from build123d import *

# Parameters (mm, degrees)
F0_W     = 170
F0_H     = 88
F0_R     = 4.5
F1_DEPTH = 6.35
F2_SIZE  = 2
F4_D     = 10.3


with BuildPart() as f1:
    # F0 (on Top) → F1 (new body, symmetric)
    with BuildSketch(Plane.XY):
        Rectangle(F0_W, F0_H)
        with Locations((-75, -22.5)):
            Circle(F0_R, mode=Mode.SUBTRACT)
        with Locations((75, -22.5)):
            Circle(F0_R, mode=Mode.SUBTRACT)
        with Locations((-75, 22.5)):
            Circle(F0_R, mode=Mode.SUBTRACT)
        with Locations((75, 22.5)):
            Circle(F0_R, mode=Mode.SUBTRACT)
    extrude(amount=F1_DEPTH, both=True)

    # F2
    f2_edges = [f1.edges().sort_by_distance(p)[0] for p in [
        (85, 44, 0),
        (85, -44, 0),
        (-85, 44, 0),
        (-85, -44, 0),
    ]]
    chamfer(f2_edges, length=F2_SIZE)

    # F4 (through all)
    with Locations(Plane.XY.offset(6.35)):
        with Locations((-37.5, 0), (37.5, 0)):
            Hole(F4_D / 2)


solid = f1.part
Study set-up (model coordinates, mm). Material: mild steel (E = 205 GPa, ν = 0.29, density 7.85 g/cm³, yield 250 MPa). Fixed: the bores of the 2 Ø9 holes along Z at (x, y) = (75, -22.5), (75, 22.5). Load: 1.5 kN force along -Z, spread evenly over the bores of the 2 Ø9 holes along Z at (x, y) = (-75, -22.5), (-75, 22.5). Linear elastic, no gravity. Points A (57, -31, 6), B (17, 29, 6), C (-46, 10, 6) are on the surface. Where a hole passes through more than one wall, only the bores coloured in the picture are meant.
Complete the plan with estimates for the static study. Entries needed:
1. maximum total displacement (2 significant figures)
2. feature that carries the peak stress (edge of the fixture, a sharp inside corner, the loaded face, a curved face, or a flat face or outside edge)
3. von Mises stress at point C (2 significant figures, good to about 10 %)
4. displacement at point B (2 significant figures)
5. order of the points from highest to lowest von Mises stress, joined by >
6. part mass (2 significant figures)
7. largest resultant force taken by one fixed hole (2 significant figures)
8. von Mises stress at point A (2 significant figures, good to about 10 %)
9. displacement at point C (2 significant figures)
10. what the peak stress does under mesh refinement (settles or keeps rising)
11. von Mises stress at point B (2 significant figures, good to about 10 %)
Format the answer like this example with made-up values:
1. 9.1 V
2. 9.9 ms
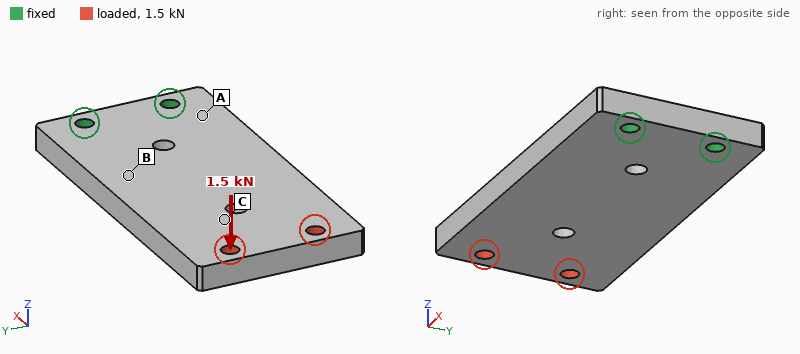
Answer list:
1. 0.63 mm
2. edge of the fixture
3. 21 MPa
4. 0.12 mm
5. A > B > C
6. 1.4 kg
7. 750 N
8. 82 MPa
9. 0.41 mm
10. keeps rising
11. 59 MPa
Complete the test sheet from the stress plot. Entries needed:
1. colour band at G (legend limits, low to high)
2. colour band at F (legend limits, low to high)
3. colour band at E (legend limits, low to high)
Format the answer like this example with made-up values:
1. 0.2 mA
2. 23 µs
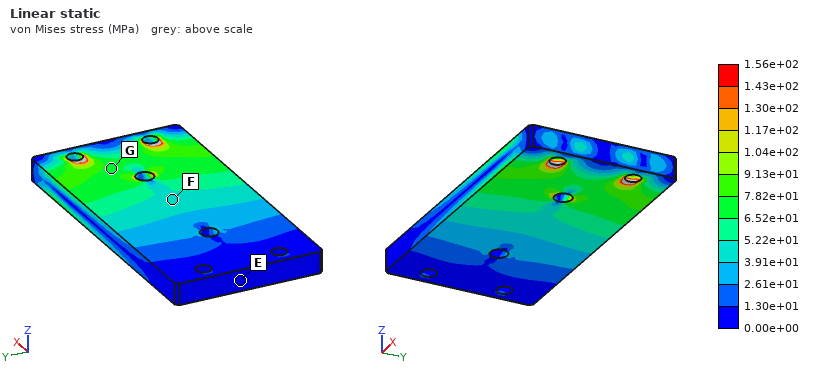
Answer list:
1. 6.52e+01 to 7.82e+01 MPa
2. 3.91e+01 to 5.22e+01 MPa
3. 0.00e+00 to 1.30e+01 MPa
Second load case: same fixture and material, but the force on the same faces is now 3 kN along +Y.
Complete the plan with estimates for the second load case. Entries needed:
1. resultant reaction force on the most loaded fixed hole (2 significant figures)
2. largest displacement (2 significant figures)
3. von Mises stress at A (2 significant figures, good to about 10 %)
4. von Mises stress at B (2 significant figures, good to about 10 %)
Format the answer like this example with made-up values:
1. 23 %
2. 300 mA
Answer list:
1. 8.8 kN
2. 44 µm
3. 20 MPa
4. 12 MPa
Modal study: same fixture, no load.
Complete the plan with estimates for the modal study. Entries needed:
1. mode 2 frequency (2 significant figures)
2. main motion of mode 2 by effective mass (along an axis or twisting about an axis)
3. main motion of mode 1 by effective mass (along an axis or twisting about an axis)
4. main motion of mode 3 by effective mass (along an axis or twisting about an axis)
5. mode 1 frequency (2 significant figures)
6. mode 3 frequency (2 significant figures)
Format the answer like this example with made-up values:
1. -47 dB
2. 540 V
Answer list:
1. 1500 Hz
2. twisting about X
3. along Z
4. along Y
5. 410 Hz
6. 2000 Hz
